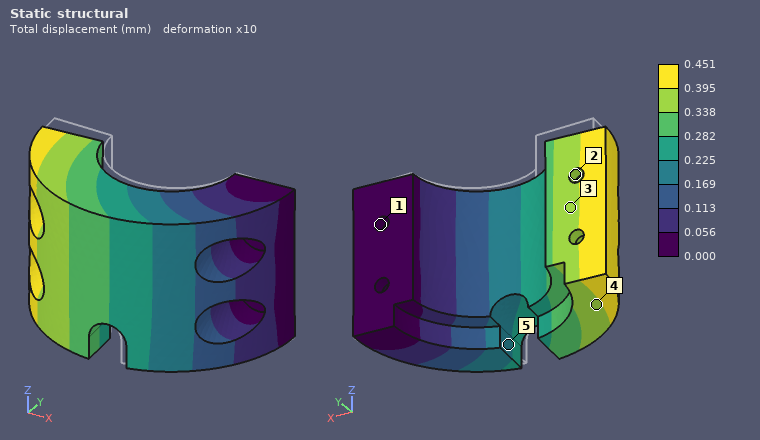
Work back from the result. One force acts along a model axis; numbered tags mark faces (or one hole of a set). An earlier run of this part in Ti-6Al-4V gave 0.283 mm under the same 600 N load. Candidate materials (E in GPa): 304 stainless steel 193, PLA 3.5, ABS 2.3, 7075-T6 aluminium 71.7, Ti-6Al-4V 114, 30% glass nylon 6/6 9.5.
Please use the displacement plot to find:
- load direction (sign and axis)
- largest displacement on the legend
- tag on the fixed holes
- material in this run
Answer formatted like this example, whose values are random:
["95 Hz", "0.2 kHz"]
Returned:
["-Y", "0.451 mm", "1", "7075-T6 aluminium"]
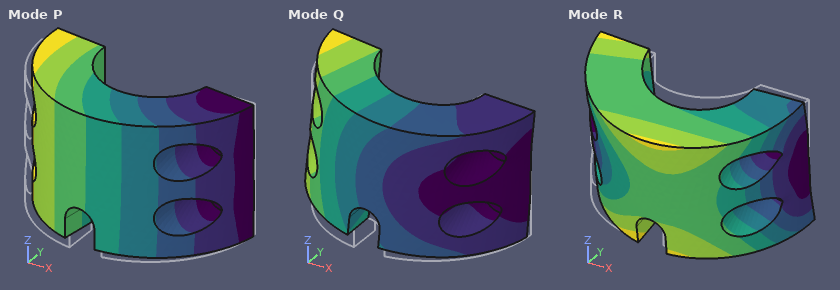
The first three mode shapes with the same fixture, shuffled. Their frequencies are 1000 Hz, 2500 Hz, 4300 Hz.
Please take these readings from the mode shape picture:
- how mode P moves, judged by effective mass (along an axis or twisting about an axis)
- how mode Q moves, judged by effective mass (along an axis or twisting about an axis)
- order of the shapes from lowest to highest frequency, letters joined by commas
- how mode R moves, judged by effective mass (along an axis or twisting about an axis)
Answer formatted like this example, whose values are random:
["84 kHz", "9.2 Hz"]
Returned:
["along Y", "along Z", "P, Q, R", "along Z"]
